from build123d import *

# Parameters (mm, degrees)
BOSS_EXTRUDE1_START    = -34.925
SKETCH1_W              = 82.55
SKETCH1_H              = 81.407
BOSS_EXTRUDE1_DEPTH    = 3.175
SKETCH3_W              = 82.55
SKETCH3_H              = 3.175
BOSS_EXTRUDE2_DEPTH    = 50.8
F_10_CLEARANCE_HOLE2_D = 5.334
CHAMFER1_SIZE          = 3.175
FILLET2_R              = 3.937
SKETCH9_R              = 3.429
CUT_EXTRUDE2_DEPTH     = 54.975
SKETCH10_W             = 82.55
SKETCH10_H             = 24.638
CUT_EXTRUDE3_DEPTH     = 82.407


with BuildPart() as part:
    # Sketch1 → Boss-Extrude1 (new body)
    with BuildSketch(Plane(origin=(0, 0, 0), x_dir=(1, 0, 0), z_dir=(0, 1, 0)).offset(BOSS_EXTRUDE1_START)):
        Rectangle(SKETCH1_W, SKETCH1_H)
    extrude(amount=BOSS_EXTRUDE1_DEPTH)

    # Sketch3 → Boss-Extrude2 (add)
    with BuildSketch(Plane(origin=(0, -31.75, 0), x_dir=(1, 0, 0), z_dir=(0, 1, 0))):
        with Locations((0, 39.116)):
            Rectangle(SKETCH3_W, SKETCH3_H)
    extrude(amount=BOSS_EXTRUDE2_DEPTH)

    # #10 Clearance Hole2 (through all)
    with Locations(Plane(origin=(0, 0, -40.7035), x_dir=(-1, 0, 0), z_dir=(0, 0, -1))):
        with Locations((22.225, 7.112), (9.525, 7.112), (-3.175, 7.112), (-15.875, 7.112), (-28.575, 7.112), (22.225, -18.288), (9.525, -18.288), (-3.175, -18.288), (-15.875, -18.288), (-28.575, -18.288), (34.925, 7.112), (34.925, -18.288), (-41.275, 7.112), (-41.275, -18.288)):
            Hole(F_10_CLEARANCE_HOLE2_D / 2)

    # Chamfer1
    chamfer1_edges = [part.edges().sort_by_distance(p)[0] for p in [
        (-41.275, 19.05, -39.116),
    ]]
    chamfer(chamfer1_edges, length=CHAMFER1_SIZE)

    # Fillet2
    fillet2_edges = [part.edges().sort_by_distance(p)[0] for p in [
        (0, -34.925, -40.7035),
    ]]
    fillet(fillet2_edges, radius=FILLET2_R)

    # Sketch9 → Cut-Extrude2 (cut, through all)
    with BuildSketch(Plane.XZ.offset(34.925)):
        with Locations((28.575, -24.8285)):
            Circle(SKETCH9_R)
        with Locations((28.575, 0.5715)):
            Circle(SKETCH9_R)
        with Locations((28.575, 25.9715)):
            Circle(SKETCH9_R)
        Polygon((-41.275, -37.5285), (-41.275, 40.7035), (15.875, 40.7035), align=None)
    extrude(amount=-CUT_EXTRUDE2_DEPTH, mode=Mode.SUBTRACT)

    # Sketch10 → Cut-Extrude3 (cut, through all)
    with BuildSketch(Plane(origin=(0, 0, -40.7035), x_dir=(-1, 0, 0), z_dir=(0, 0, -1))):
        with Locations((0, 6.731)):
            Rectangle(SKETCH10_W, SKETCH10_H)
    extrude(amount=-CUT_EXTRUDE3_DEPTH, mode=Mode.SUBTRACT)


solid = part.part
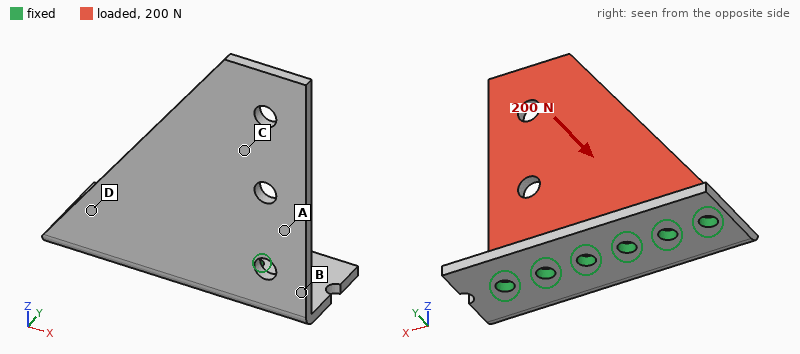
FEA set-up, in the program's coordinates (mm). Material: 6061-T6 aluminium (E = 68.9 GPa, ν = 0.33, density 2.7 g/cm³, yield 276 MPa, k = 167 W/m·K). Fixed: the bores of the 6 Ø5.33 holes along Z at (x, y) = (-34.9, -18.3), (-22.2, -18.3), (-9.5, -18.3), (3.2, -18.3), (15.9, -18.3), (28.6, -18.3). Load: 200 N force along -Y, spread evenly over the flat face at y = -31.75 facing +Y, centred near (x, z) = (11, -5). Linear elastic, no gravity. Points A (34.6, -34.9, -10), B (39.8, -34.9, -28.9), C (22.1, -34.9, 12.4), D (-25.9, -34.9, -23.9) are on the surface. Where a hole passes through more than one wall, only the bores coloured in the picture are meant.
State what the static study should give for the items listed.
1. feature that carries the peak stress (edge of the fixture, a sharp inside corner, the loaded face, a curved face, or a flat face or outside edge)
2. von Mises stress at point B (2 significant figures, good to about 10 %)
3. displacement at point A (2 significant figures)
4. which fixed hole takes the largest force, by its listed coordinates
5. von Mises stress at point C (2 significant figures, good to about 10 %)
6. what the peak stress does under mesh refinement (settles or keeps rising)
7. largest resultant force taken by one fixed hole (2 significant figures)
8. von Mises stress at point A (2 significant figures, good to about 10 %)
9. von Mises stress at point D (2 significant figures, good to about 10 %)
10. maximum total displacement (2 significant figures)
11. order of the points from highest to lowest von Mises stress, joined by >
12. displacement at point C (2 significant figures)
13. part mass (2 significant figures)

edge of the fixture
49 MPa
0.38 mm
(28.6, -18.3)
11 MPa
keeps rising
63 N
22 MPa
35 MPa
1.4 mm
B > D > A > C
0.76 mm
54 g
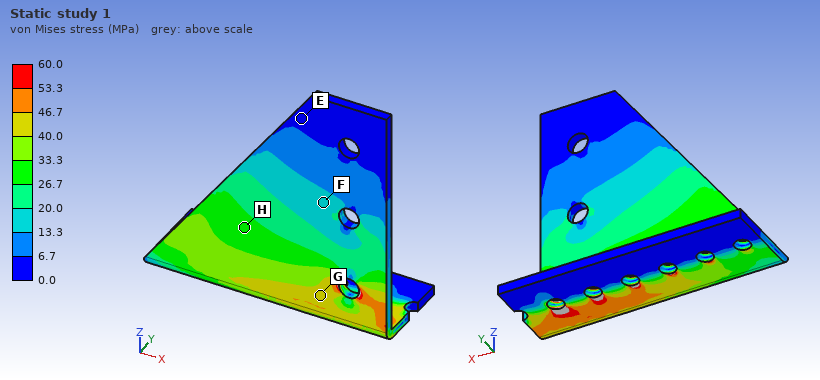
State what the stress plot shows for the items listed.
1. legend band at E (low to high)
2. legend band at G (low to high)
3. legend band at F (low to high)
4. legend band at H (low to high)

0.0 to 6.7 MPa
40.0 to 46.7 MPa
13.3 to 20.0 MPa
26.7 to 33.3 MPa
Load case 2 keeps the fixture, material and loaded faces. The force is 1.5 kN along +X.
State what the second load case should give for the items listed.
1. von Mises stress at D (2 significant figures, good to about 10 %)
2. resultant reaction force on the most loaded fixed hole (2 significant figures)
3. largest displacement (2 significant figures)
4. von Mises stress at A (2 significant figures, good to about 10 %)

20 MPa
710 N
0.65 mm
21 MPa
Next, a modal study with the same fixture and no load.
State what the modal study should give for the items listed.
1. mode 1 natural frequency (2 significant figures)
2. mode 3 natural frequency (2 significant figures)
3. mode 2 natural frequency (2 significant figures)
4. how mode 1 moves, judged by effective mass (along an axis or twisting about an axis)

430 Hz
2000 Hz
1700 Hz
along Y
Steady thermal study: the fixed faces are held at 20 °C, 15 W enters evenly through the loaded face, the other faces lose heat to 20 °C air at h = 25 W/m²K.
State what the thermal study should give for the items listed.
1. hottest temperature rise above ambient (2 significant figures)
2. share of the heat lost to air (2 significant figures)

19 K
12 %
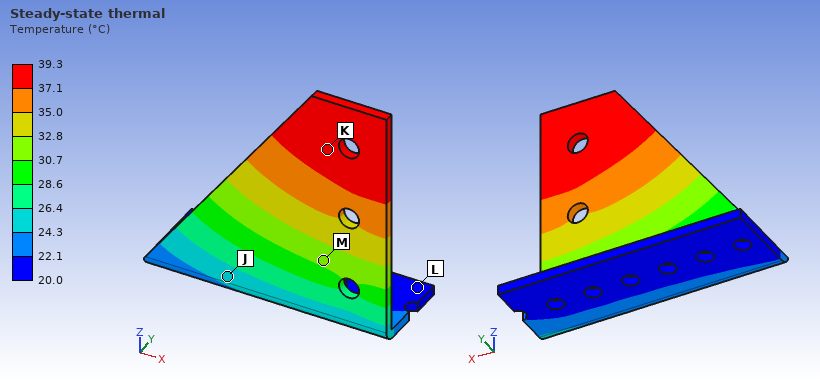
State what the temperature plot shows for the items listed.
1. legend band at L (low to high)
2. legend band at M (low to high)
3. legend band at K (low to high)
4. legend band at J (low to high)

20.0 to 22.1 °C
30.7 to 32.8 °C
37.1 to 39.3 °C
24.3 to 26.4 °C
